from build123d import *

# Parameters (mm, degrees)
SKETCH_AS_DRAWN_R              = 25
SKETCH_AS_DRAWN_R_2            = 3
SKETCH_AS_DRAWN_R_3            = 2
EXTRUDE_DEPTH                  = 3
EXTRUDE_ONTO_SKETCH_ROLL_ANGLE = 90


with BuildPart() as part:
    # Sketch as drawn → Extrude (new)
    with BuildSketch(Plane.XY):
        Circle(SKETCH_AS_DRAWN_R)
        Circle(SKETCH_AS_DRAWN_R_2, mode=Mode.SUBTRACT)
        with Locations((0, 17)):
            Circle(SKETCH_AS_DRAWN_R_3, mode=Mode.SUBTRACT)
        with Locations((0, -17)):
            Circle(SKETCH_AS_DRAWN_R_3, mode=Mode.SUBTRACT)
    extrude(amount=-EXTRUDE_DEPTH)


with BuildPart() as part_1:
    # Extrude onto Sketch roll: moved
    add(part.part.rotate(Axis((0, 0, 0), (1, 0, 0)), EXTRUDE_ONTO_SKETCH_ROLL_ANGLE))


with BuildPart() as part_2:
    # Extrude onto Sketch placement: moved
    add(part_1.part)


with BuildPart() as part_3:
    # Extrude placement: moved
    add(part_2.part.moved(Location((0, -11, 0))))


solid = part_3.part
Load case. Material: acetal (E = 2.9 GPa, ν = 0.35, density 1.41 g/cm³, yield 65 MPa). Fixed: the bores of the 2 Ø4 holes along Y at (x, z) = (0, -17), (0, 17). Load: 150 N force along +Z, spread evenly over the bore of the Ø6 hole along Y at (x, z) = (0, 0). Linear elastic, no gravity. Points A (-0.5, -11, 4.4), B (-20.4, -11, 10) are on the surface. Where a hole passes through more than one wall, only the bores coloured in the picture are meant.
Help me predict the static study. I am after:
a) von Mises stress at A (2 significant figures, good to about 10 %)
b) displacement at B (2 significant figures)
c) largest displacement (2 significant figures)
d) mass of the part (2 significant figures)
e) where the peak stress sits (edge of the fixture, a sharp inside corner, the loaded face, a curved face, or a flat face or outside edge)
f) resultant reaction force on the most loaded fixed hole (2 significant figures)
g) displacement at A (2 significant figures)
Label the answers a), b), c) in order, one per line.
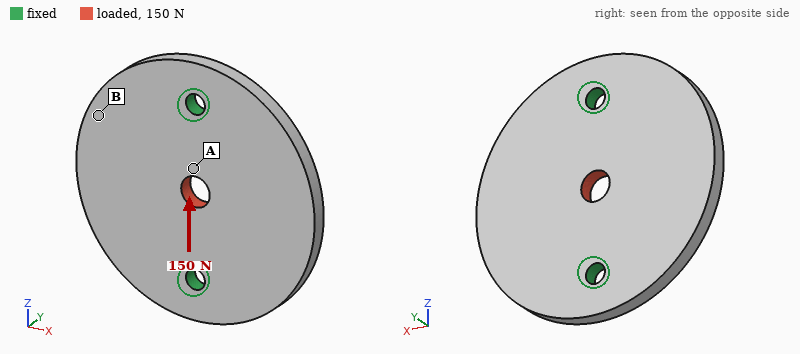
a) 2.7 MPa
b) 4.8 µm
c) 11 µm
d) 8.1 g
e) the loaded face
f) 75 N
g) 9.4 µm
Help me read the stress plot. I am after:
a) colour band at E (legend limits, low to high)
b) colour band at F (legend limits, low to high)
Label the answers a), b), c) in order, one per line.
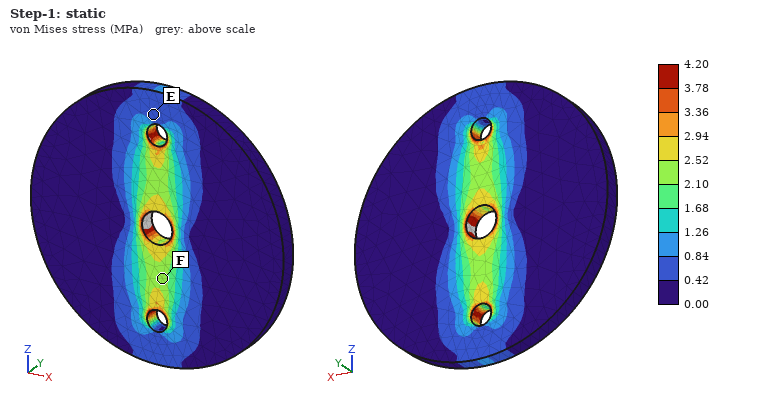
a) 0.42 to 0.84 MPa
b) 2.10 to 2.52 MPa
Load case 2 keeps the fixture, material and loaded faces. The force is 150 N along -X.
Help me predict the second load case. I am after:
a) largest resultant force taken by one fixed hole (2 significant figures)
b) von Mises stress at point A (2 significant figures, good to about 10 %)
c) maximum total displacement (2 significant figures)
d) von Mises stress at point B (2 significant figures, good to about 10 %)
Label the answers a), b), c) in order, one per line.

a) 75 N
b) 2.1 MPa
c) 16 µm
d) 0.69 MPa
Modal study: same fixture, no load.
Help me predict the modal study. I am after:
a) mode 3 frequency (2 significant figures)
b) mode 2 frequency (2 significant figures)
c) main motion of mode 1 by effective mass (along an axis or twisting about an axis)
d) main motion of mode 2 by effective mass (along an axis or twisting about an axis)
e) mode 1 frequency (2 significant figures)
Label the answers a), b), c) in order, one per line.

a) 2900 Hz
b) 1400 Hz
c) twisting about Z
d) along Y
e) 1200 Hz
